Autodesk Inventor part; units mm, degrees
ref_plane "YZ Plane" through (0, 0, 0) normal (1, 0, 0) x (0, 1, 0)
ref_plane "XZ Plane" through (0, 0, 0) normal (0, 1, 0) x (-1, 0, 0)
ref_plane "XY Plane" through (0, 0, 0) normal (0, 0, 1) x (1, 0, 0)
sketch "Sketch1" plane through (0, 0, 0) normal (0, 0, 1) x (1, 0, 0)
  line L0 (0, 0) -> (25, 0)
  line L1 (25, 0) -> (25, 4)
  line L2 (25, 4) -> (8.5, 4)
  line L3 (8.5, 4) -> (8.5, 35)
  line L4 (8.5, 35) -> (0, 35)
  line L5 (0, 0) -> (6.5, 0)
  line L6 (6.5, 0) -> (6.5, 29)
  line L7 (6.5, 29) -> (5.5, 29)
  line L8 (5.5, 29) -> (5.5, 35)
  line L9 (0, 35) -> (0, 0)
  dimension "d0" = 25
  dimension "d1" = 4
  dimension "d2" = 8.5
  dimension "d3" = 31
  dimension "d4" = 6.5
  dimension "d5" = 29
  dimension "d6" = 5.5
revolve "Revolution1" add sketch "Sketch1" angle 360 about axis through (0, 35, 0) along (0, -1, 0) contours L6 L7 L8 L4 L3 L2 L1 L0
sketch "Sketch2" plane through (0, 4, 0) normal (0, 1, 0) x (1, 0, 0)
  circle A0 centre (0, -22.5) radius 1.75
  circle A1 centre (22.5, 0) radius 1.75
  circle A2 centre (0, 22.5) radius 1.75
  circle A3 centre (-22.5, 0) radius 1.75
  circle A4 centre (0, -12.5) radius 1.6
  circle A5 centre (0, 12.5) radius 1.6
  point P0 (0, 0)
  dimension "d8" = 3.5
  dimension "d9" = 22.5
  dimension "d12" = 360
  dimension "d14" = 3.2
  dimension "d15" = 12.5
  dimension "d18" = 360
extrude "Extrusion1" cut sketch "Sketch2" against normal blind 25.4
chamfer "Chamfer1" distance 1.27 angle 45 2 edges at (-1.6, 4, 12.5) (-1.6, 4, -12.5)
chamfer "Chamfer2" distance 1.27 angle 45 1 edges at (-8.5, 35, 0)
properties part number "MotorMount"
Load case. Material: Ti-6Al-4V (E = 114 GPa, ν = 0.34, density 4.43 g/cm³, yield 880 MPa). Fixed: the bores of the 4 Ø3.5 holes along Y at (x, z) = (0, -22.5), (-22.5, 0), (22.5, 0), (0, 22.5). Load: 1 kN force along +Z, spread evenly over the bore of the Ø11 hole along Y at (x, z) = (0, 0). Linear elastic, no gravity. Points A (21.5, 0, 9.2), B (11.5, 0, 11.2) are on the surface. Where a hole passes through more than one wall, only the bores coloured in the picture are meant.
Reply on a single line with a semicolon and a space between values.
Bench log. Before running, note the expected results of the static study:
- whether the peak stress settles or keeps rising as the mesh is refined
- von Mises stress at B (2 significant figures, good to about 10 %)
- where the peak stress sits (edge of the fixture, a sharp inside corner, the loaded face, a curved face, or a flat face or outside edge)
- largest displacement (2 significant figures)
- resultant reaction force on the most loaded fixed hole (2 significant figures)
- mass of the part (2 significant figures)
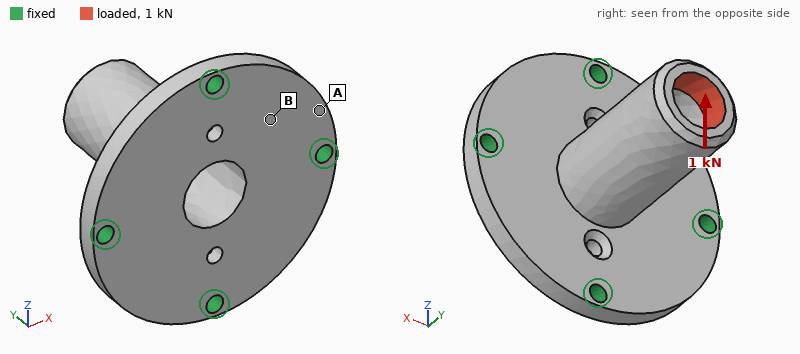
keeps rising; 46 MPa; edge of the fixture; 0.14 mm; 870 N; 45 g
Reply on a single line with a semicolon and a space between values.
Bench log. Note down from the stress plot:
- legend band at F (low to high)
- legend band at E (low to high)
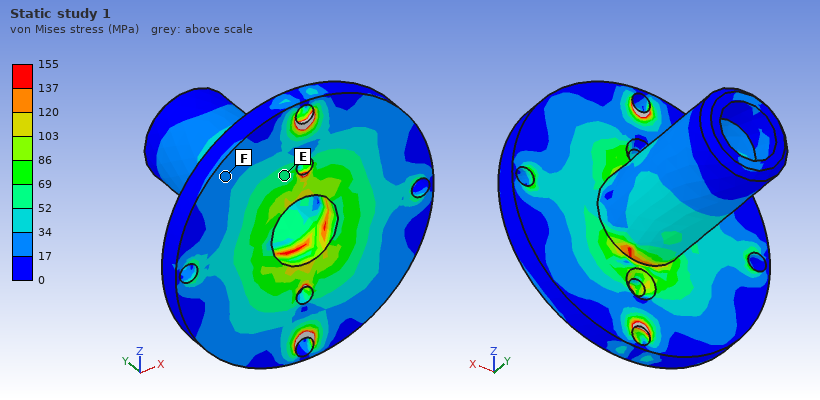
17 to 34 MPa; 52 to 69 MPa
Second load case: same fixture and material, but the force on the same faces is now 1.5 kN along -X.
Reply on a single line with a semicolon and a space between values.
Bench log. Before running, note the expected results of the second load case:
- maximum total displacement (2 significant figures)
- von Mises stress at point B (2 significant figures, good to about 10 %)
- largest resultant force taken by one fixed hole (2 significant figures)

0.20 mm; 67 MPa; 1.3 kN
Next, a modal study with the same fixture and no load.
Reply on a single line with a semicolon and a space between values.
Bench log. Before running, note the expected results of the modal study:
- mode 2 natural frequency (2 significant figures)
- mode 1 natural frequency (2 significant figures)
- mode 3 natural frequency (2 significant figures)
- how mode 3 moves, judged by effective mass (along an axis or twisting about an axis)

5700 Hz; 5600 Hz; 9800 Hz; along Y
